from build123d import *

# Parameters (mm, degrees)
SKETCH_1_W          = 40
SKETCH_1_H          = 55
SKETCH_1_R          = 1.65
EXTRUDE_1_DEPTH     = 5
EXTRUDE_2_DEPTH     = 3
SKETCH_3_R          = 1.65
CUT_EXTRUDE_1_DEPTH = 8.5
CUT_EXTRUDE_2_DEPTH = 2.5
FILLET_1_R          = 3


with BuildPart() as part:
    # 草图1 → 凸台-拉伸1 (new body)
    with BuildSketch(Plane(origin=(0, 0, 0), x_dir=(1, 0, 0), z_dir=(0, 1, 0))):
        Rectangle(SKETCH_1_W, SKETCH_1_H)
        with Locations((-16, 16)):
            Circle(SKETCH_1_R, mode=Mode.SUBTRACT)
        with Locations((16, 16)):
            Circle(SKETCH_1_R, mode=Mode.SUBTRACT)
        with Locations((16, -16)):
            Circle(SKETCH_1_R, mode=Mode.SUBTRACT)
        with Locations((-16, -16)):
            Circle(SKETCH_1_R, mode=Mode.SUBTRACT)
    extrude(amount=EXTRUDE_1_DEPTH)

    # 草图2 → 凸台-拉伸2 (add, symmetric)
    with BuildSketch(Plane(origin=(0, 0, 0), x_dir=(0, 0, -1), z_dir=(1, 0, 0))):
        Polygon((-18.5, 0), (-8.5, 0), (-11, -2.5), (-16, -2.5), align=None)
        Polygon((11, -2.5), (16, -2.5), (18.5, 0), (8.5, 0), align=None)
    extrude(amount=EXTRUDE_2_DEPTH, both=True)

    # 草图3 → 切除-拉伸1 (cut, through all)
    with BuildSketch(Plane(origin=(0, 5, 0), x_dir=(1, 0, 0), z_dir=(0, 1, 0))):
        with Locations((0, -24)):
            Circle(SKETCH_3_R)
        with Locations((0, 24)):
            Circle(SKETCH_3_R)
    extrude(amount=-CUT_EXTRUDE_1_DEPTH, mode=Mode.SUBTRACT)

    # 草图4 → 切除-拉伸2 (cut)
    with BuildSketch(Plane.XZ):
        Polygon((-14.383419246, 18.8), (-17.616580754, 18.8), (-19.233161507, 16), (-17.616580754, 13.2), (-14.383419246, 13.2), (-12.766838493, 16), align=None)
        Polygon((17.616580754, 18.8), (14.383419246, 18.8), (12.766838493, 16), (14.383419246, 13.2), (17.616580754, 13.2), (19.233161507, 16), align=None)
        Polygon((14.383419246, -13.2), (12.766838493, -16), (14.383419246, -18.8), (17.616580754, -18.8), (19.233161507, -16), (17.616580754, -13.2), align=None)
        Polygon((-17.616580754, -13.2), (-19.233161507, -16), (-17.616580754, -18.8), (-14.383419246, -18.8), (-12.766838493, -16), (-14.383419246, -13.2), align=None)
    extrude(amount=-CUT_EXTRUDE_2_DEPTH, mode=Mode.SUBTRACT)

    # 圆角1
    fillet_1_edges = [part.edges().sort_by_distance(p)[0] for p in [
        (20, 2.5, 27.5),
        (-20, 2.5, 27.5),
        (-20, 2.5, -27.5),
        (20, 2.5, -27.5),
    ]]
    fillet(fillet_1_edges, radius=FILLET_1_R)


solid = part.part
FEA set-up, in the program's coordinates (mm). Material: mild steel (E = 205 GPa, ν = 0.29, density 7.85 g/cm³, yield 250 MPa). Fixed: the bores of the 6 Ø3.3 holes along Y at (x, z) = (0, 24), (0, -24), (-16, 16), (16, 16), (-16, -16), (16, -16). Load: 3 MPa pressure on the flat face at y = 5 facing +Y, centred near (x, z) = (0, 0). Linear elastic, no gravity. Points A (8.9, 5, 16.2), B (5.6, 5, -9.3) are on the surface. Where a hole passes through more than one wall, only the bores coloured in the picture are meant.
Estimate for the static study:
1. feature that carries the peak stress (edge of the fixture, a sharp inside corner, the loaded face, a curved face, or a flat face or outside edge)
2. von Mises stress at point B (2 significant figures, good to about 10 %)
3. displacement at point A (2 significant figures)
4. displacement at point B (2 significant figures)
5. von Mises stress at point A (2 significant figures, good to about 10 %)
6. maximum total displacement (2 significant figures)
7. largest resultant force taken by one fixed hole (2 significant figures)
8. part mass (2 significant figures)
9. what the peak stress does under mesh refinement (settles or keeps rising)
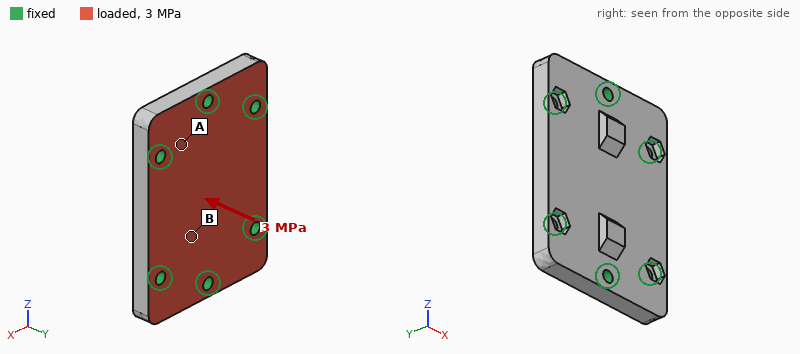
edge of the fixture
17 MPa
3.2 µm
8.1 µm
32 MPa
12 µm
1.2 kN
84 g
keeps rising
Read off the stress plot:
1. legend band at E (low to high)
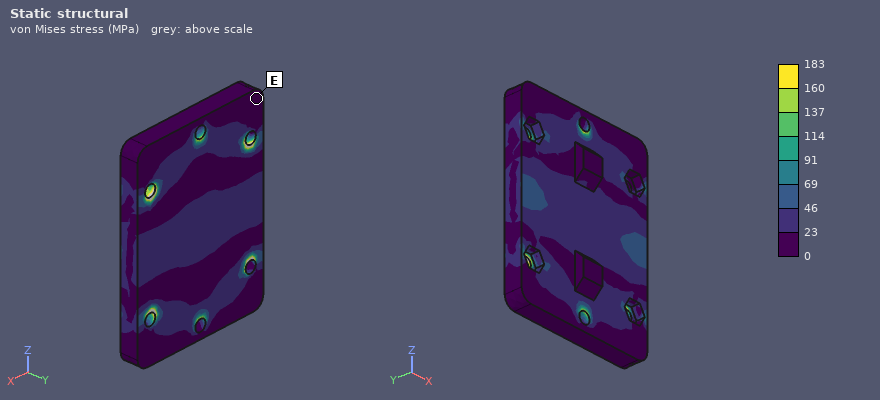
0 to 23 MPa
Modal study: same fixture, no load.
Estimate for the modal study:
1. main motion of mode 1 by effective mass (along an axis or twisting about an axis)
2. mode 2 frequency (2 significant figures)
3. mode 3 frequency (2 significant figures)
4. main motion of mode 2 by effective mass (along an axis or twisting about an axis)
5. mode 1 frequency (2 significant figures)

along Y
21 kHz
29 kHz
twisting about Z
15 kHz
